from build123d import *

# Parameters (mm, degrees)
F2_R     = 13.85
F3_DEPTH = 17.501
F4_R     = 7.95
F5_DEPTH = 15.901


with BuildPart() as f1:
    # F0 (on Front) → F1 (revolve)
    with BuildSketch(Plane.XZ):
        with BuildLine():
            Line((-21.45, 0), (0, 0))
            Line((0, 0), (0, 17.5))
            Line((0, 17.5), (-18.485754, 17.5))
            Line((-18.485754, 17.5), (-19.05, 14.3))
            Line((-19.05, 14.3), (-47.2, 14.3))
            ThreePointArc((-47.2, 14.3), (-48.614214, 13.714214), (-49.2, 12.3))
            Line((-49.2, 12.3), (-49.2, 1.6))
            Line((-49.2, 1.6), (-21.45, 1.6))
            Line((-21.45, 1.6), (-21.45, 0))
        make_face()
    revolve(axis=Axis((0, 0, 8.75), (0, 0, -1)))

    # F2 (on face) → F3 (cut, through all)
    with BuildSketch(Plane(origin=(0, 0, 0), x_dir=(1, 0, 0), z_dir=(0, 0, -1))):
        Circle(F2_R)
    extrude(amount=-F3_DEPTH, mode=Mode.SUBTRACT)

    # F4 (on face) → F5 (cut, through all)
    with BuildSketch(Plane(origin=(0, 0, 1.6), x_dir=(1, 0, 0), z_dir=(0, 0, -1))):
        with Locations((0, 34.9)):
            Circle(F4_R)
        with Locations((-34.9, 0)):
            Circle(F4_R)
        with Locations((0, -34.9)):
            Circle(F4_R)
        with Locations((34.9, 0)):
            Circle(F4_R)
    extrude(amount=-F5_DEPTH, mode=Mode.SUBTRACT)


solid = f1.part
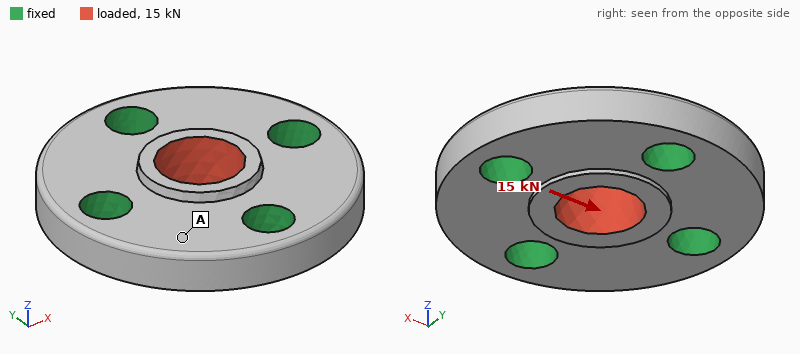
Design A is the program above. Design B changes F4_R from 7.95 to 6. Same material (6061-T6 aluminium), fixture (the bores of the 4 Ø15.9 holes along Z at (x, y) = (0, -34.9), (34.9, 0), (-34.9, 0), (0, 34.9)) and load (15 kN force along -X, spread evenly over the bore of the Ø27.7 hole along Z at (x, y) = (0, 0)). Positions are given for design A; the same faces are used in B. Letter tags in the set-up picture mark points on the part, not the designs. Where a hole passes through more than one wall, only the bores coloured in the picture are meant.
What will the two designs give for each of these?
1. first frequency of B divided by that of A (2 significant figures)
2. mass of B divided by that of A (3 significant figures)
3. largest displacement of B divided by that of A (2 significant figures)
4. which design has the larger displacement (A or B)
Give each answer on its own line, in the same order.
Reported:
0.85
1.05
1.1
B
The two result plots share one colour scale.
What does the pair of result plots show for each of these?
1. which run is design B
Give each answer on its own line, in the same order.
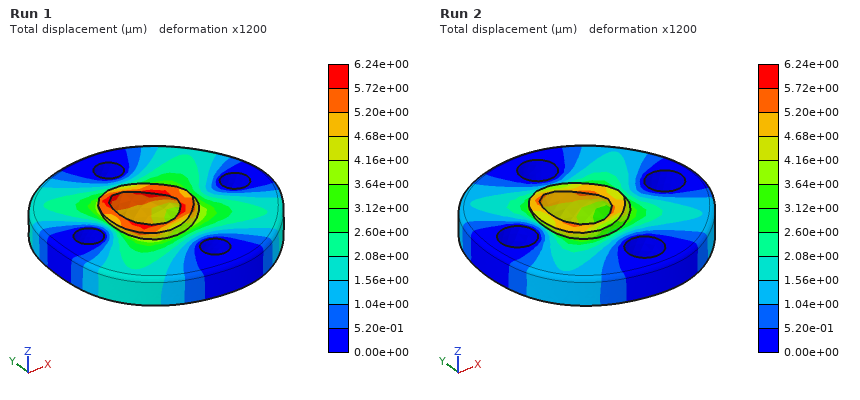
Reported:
Run 1
